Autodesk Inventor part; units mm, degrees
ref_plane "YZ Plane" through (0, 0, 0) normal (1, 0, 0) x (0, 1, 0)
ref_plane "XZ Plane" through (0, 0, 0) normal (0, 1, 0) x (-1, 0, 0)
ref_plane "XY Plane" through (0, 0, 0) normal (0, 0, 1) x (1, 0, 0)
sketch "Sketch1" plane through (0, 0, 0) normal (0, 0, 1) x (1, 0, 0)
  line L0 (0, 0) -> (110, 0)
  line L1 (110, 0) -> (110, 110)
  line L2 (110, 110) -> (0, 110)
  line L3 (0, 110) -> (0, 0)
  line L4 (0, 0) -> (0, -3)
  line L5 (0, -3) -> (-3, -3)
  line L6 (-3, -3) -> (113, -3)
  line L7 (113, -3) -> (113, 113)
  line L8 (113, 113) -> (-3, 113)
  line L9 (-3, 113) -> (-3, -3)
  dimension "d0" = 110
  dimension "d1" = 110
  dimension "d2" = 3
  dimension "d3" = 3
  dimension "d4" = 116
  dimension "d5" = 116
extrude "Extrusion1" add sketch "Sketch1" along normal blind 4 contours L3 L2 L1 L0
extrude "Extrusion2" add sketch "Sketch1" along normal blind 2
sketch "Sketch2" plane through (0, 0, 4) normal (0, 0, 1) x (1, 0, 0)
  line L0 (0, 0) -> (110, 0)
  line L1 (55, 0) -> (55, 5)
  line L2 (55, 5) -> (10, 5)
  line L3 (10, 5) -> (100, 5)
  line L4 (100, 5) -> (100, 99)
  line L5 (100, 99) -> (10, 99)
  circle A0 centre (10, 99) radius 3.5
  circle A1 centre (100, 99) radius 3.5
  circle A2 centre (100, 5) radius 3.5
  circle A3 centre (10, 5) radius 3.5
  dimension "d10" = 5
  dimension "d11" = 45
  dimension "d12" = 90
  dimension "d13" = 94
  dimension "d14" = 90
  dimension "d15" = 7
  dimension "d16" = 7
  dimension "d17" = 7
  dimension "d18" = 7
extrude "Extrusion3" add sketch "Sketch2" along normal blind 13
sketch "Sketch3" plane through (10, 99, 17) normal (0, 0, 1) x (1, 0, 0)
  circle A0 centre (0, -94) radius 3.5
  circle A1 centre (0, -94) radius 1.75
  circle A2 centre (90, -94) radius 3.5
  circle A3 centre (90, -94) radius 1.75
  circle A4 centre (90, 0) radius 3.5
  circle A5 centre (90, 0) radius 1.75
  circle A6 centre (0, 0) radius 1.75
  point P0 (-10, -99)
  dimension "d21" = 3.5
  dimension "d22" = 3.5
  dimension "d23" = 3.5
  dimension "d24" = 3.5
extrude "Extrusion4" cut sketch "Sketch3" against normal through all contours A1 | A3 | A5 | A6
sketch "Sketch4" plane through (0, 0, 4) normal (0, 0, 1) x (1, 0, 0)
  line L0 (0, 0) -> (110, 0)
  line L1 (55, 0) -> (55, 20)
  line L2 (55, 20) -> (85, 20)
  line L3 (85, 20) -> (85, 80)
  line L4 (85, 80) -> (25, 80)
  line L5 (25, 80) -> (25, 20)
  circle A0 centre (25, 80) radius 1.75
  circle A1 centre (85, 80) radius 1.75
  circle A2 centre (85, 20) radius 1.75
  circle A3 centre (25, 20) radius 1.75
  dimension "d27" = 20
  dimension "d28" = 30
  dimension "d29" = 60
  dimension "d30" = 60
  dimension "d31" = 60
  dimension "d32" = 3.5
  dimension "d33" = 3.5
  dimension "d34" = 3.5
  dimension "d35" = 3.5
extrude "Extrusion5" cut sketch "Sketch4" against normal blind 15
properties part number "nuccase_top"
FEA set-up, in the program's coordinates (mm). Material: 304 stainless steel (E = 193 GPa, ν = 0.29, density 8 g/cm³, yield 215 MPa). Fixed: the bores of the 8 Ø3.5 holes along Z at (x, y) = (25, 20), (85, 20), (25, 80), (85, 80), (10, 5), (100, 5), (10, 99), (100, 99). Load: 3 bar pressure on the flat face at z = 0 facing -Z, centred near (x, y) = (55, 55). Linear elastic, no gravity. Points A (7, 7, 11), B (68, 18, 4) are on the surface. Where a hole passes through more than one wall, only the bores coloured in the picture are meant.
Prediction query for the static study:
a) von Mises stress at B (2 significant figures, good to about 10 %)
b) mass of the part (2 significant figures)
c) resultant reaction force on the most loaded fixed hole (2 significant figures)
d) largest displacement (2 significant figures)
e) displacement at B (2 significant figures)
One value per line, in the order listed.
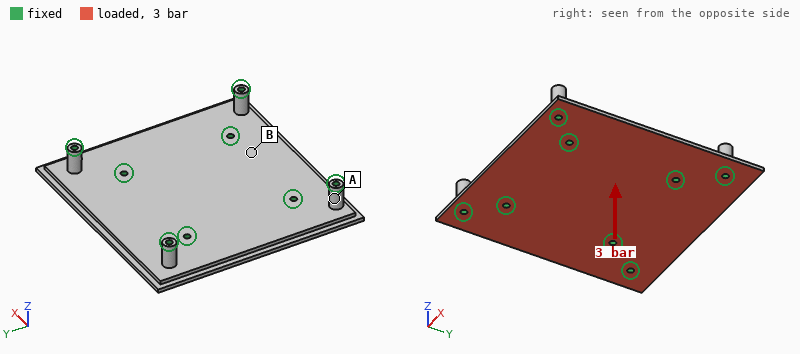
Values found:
18 MPa
420 g
800 N
34 µm
10 µm
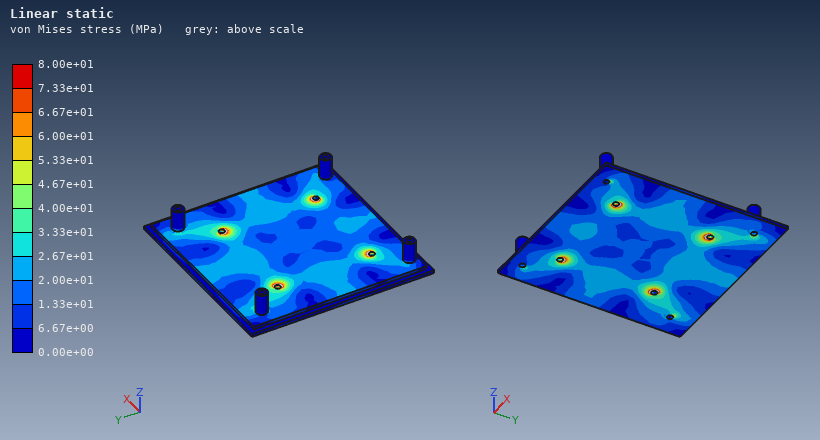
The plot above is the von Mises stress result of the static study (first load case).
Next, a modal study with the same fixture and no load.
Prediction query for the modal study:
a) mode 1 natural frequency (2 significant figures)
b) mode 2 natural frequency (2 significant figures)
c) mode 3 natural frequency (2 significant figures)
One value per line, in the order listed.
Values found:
3400 Hz
3800 Hz
3800 Hz
